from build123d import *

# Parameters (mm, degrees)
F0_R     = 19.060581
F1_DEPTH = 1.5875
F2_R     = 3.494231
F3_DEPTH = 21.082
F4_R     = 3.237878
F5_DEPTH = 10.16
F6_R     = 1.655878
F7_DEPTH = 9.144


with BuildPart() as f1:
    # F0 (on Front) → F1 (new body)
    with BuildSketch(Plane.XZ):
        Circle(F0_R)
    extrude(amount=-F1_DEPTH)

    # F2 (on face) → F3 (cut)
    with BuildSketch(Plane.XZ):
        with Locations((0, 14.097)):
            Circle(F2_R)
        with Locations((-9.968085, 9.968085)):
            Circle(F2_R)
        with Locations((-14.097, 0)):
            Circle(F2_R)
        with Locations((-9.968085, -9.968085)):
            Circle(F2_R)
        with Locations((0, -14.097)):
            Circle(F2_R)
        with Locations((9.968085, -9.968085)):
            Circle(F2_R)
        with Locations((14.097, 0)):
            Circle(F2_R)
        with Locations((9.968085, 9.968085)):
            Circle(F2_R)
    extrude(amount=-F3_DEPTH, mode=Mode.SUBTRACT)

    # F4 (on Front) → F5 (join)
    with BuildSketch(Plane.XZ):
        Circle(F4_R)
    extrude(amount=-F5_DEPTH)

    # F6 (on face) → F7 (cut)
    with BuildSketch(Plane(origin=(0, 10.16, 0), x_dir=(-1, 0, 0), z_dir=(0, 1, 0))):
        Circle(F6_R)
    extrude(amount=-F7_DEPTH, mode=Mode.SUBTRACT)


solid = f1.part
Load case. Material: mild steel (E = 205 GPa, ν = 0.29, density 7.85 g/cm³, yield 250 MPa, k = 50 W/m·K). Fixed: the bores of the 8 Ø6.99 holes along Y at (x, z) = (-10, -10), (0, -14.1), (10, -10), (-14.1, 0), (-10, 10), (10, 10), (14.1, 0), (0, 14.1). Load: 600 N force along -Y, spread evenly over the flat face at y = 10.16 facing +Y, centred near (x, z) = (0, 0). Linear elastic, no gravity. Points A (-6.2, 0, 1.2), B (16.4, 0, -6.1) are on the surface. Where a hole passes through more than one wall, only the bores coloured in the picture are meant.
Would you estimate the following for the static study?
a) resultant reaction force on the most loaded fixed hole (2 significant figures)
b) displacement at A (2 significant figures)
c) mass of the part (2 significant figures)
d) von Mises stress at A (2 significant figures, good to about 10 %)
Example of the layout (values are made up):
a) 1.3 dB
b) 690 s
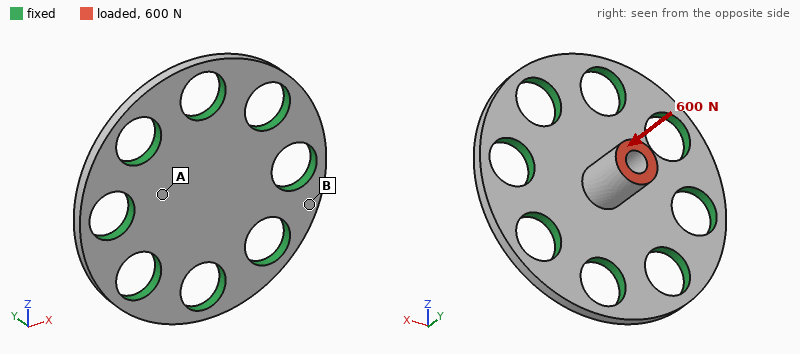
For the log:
a) 79 N
b) 5.6 µm
c) 12 g
d) 46 MPa
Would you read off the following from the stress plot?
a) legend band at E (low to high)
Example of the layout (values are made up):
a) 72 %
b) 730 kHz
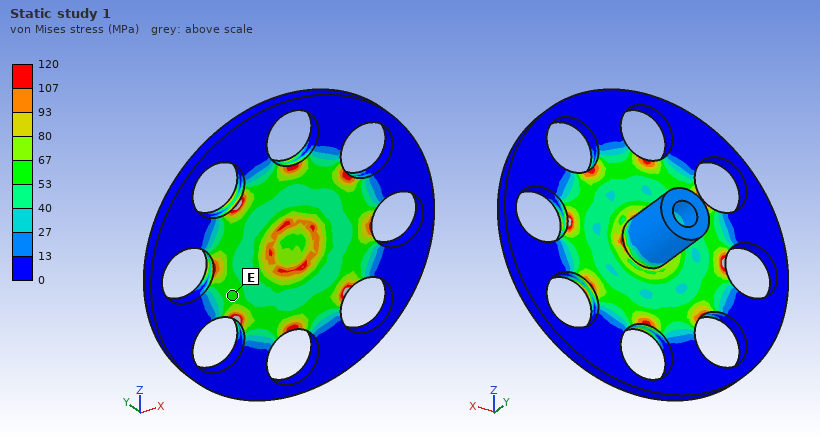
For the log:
a) 53 to 67 MPa
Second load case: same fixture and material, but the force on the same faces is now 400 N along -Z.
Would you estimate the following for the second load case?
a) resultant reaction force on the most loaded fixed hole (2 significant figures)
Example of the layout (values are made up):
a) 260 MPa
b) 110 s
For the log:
a) 150 N
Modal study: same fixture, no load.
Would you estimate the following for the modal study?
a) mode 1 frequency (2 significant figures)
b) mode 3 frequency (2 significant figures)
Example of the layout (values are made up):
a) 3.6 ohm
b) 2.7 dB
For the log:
a) 21 kHz
b) 22 kHz
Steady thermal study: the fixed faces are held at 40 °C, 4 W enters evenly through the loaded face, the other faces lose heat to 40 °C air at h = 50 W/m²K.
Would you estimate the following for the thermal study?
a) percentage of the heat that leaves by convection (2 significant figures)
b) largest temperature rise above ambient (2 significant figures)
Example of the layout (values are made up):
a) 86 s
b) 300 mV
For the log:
a) 11 %
b) 38 K
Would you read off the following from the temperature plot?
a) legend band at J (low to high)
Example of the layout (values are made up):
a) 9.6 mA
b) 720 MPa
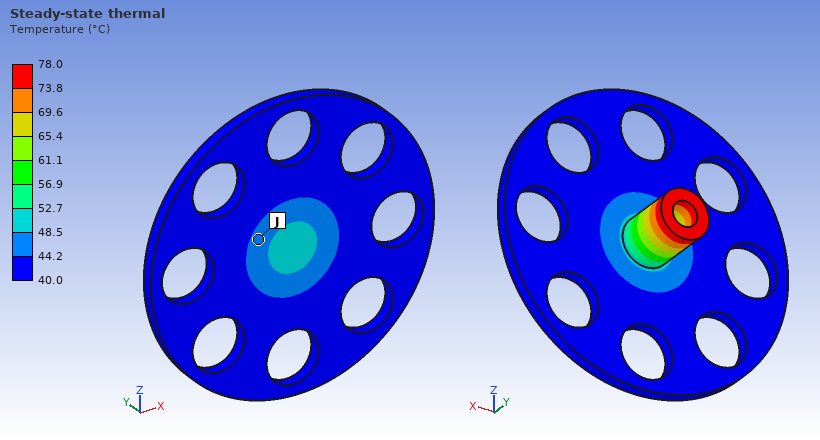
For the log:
a) 44.2 to 48.5 °C
